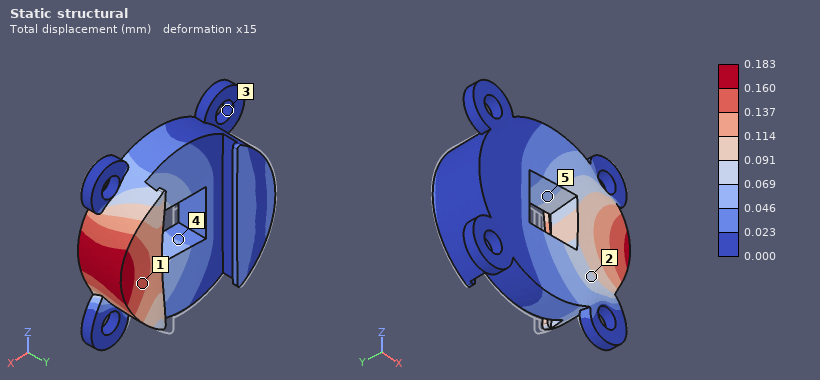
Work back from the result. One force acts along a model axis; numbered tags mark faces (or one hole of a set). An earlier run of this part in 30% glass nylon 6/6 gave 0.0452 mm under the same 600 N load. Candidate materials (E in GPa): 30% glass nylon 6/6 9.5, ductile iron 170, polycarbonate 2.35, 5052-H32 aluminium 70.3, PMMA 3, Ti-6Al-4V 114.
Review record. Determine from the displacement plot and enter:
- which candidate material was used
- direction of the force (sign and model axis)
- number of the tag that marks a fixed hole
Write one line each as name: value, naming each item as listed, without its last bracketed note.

which candidate material was used: polycarbonate
direction of the force: -Y
number of the tag that marks a fixed hole: 3
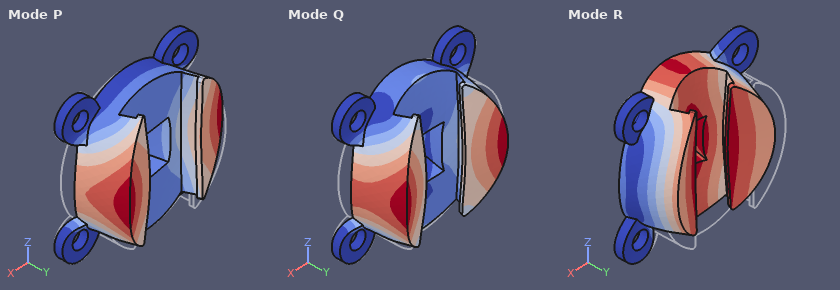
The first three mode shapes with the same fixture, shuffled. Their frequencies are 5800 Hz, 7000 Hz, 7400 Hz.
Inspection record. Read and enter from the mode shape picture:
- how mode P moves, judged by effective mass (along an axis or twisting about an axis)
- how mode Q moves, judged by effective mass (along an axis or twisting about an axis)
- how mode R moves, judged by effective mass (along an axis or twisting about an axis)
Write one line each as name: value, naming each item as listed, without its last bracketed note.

how mode P moves, judged by effective mass: along X
how mode Q moves, judged by effective mass: along Y
how mode R moves, judged by effective mass: along Y
